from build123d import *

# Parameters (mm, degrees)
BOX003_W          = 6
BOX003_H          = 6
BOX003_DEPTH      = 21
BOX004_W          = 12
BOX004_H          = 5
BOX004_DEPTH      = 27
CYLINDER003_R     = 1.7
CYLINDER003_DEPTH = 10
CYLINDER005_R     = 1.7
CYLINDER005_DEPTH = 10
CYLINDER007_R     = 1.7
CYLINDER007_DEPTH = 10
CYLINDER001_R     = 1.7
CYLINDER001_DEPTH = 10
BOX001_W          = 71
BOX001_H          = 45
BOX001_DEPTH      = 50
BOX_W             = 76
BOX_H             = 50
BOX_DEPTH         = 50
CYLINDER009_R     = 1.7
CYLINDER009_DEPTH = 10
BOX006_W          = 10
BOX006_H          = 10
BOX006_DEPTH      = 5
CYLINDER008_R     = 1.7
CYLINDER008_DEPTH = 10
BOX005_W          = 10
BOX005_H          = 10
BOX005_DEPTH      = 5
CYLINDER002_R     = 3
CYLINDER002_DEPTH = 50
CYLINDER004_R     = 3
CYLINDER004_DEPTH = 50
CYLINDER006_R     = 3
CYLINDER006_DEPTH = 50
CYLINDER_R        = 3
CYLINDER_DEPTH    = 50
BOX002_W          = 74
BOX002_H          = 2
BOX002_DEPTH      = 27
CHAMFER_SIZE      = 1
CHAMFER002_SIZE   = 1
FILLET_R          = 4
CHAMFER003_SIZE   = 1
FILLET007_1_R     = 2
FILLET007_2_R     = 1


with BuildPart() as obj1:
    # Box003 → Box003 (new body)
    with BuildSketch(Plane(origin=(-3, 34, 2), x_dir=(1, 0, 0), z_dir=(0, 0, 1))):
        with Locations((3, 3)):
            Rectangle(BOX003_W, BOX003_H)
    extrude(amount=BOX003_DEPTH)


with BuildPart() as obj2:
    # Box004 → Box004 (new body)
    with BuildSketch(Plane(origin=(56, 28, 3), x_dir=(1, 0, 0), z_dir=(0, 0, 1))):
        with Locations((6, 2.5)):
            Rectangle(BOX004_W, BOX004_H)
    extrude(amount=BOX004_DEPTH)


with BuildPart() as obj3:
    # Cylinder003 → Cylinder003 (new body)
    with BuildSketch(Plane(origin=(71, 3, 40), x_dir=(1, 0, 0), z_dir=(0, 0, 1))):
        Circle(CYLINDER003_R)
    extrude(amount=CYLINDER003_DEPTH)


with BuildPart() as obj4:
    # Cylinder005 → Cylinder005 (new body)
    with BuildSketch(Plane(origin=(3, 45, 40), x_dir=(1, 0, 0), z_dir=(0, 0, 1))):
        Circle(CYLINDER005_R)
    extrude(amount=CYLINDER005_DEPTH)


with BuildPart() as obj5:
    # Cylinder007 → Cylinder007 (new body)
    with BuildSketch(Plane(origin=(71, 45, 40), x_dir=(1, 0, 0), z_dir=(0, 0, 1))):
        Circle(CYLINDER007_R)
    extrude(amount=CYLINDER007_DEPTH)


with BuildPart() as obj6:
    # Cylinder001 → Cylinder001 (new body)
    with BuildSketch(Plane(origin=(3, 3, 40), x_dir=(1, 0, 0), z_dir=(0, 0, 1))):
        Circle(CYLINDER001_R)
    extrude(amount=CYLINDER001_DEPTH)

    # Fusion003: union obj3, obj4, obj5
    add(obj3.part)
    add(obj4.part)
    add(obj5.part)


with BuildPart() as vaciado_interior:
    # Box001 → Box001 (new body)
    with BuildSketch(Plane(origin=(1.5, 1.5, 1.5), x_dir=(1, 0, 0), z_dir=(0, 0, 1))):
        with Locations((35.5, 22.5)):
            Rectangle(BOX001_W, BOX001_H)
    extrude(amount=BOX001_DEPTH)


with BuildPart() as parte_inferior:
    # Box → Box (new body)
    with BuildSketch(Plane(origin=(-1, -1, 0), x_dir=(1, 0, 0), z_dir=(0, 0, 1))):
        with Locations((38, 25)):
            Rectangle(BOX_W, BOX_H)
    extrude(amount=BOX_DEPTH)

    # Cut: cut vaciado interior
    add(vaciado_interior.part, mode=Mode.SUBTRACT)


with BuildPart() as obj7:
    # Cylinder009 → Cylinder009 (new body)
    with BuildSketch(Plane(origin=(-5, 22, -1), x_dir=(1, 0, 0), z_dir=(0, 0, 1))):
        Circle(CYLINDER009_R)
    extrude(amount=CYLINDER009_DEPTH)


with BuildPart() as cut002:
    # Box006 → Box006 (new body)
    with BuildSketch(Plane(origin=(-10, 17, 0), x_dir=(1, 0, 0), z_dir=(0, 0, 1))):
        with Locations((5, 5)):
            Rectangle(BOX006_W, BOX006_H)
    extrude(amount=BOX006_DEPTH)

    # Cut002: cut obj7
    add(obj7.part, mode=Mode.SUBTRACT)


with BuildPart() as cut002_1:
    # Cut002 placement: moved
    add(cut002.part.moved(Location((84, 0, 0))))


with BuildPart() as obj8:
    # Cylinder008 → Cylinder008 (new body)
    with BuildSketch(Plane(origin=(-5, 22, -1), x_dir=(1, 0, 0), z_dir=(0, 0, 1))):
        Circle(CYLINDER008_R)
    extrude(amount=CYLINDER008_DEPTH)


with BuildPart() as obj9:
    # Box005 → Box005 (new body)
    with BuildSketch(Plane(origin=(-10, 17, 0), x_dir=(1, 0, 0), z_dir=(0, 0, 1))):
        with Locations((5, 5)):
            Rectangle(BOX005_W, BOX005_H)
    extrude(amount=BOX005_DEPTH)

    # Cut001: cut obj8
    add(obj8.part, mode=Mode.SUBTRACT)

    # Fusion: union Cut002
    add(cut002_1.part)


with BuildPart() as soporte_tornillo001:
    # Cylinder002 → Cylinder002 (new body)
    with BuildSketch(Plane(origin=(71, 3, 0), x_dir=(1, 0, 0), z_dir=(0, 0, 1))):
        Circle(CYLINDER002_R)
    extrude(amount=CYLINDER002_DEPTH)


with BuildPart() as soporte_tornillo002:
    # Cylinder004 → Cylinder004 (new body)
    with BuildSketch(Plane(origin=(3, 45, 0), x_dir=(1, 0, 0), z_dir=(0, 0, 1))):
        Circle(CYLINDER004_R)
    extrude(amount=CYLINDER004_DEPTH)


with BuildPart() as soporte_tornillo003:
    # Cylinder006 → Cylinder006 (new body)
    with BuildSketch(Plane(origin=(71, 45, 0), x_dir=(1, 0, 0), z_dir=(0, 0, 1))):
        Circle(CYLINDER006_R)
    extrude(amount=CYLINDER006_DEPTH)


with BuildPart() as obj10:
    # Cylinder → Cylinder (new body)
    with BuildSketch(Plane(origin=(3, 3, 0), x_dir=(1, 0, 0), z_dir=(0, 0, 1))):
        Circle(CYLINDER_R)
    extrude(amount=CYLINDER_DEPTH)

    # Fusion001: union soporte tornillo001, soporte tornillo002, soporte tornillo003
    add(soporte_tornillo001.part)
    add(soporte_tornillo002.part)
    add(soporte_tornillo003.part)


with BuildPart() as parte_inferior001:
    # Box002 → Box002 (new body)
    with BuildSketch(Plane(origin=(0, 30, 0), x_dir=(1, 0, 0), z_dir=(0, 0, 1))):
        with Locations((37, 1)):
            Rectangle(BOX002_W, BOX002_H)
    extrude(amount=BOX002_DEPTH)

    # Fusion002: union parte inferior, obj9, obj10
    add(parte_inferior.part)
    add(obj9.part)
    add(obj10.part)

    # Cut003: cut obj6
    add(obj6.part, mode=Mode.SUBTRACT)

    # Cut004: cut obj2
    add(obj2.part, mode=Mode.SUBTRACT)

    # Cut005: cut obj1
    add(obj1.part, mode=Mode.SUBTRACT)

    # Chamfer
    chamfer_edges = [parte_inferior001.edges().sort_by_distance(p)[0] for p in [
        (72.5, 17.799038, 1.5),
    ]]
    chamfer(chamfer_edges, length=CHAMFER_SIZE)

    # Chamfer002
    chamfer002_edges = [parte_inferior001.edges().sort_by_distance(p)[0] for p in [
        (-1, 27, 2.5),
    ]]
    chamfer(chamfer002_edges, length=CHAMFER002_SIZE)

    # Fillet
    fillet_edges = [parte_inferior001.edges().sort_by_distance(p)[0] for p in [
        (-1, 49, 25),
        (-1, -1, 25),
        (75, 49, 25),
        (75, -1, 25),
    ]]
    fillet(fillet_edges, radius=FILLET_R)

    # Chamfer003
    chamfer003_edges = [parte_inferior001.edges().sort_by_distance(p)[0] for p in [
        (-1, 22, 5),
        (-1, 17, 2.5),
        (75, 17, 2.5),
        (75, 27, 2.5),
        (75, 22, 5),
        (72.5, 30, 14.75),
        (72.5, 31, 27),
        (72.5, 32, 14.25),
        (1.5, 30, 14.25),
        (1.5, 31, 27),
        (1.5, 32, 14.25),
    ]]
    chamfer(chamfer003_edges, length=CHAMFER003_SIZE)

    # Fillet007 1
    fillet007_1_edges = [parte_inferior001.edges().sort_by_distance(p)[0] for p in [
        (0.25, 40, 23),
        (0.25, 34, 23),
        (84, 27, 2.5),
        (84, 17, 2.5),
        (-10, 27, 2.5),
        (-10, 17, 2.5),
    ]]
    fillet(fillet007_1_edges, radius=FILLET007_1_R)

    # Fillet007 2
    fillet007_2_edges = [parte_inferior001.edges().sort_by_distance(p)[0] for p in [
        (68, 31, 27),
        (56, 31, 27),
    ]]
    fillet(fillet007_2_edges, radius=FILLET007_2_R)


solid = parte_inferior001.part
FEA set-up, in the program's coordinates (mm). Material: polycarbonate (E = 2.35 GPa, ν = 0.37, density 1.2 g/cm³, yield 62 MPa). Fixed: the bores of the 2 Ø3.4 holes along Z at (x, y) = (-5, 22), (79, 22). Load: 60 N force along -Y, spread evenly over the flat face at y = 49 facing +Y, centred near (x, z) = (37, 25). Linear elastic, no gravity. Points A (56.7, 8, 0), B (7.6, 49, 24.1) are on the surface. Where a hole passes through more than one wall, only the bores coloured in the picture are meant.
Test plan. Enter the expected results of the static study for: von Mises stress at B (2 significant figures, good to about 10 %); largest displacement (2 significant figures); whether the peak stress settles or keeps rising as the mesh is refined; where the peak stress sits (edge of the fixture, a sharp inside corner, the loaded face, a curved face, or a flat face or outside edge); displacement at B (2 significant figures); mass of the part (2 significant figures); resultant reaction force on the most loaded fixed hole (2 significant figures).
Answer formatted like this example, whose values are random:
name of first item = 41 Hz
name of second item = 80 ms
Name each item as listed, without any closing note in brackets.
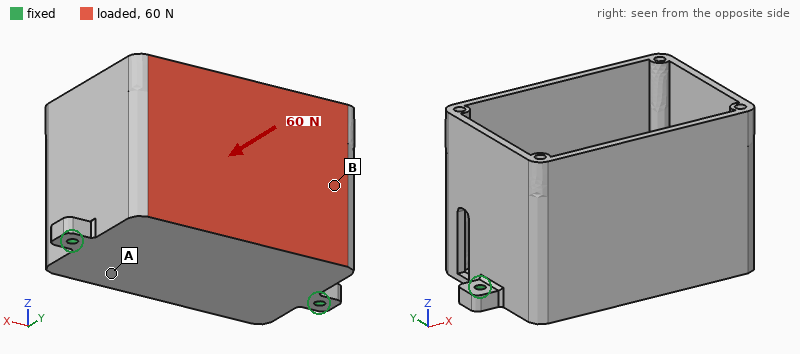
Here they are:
von Mises stress at B = 2.1 MPa
largest displacement = 1.1 mm
whether the peak stress settles or keeps rising as the mesh is refined = keeps rising
where the peak stress sits = edge of the fixture
displacement at B = 0.43 mm
mass of the part = 49 g
resultant reaction force on the most loaded fixed hole = 31 N
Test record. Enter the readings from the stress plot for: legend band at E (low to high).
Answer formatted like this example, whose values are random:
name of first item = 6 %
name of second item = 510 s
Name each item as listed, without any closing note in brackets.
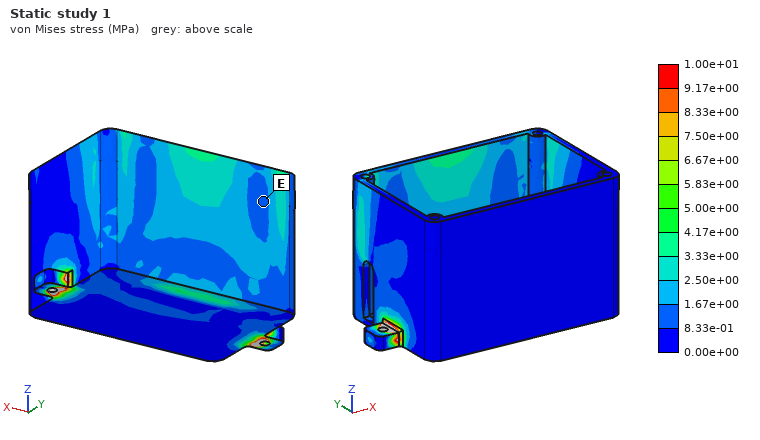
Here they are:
legend band at E = 8.33e-01 to 1.67e+00 MPa
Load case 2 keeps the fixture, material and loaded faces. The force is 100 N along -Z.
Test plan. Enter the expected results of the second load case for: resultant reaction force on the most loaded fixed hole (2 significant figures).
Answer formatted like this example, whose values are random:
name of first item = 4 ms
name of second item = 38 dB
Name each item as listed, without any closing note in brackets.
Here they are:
resultant reaction force on the most loaded fixed hole = 50 N
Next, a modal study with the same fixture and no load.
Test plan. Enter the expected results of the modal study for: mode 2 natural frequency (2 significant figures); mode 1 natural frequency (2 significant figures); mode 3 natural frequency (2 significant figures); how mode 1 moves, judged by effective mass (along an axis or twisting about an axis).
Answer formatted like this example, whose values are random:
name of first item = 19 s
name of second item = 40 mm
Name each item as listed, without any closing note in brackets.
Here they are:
mode 2 natural frequency = 440 Hz
mode 1 natural frequency = 250 Hz
mode 3 natural frequency = 680 Hz
how mode 1 moves, judged by effective mass = along Y
